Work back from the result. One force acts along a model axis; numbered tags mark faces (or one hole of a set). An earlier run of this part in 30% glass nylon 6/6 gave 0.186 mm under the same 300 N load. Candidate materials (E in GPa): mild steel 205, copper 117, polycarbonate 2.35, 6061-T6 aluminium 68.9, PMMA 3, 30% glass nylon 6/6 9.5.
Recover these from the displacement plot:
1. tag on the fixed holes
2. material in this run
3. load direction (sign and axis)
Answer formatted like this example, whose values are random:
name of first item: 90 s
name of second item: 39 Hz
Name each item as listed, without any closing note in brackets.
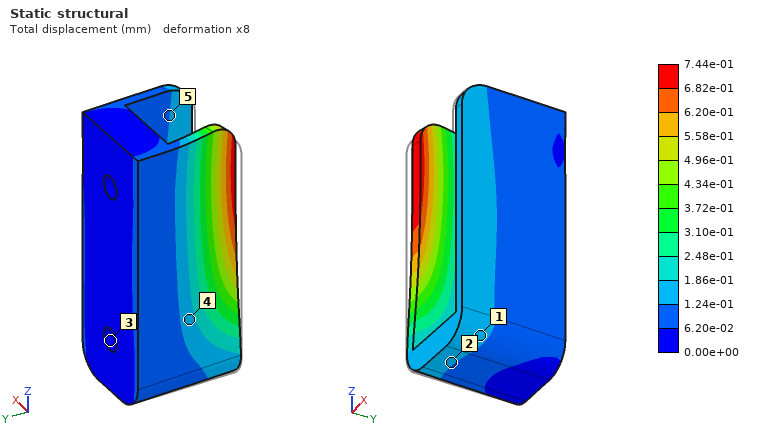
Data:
tag on the fixed holes: 3
material in this run: polycarbonate
load direction: +X
